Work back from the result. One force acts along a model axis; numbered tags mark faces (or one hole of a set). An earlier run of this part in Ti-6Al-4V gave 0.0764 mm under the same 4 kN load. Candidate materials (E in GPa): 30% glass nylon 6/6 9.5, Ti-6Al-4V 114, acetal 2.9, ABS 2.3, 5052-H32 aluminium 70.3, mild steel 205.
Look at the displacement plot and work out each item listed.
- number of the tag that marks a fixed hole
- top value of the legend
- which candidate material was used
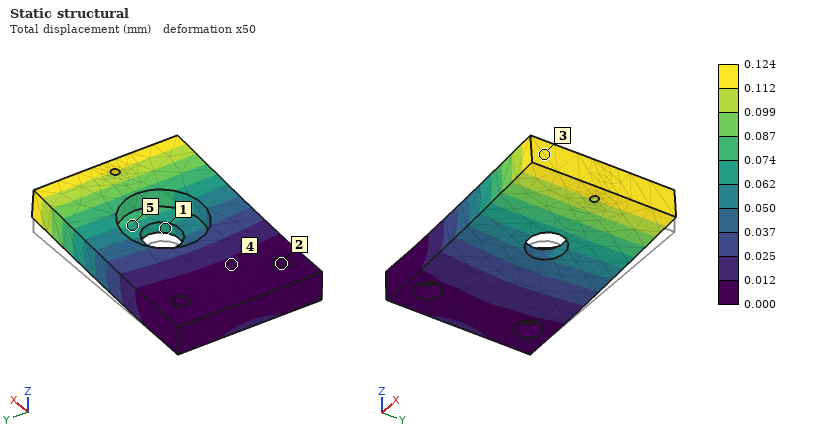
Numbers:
2
0.124 mm
5052-H32 aluminium
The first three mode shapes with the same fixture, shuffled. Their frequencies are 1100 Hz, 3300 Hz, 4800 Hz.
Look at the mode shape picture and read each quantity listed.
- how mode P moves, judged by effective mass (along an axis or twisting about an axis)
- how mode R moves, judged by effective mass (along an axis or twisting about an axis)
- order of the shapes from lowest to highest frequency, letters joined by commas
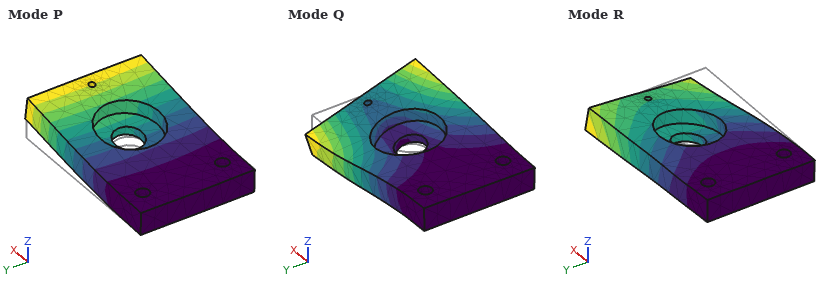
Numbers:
along Z
along Y
P, Q, R
